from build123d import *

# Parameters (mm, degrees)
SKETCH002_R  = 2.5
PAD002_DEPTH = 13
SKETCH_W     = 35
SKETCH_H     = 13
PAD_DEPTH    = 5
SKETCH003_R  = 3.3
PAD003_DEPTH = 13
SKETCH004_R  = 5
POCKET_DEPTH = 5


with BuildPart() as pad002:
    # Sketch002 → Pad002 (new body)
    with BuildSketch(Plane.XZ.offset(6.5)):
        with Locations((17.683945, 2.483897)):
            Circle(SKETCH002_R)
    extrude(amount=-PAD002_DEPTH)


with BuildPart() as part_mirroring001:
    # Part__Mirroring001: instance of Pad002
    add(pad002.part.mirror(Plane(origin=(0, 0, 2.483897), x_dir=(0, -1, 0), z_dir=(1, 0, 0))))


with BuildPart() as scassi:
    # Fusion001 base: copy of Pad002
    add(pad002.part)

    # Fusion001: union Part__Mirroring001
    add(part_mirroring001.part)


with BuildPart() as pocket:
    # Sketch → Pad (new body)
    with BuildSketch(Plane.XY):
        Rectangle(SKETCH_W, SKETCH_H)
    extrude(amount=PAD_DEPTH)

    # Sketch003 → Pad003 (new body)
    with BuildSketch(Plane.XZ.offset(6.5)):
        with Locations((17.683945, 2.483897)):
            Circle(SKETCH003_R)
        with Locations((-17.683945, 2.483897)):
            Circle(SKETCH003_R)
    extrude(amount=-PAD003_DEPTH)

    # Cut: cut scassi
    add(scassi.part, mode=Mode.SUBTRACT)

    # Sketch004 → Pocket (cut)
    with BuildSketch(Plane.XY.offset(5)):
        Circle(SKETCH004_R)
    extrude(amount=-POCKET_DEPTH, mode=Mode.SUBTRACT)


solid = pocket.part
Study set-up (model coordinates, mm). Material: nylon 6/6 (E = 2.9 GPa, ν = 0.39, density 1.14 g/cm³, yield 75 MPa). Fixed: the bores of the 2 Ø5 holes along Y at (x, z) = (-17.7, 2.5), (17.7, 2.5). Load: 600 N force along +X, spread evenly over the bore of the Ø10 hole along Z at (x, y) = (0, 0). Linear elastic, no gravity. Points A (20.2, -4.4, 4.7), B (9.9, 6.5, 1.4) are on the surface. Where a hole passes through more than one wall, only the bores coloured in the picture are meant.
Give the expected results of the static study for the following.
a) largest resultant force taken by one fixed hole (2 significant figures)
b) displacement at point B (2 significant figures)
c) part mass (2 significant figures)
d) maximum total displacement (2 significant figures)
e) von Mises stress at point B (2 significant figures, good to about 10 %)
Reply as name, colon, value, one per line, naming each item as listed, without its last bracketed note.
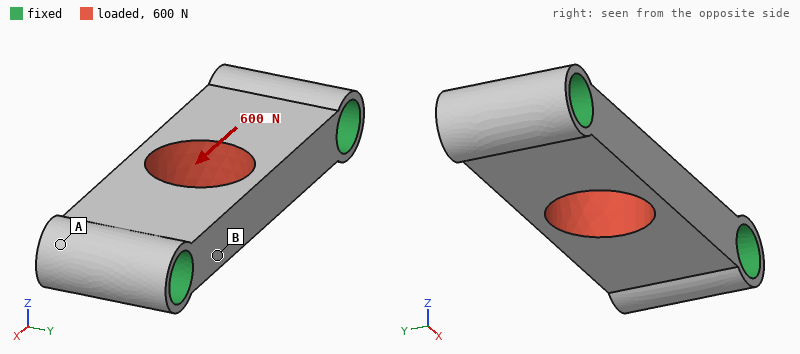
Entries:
largest resultant force taken by one fixed hole: 300 N
displacement at point B: 10 µm
part mass: 2.2 g
maximum total displacement: 27 µm
von Mises stress at point B: 4.8 MPa
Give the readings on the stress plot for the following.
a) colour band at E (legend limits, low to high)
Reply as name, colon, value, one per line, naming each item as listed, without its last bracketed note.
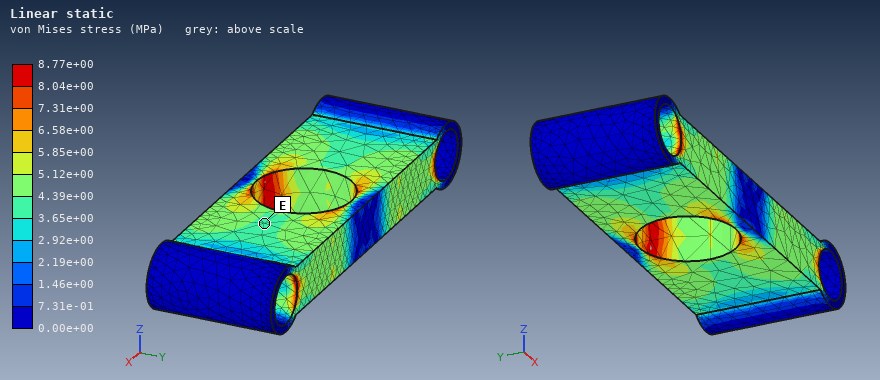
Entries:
colour band at E: 3.65e+00 to 4.39e+00 MPa
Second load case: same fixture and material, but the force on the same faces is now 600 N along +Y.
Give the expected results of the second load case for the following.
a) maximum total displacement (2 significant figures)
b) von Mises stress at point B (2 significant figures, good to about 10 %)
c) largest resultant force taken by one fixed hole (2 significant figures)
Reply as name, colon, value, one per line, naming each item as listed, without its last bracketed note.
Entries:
maximum total displacement: 0.13 mm
von Mises stress at point B: 4.8 MPa
largest resultant force taken by one fixed hole: 300 N
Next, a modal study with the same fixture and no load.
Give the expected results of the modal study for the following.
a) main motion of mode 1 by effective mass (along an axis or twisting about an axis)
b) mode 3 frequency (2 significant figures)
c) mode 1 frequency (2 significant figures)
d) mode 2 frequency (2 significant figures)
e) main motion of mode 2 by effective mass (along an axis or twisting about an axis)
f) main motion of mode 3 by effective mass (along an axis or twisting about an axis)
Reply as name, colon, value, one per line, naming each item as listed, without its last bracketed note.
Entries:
main motion of mode 1 by effective mass: along Z
mode 3 frequency: 15 kHz
mode 1 frequency: 8000 Hz
mode 2 frequency: 11 kHz
main motion of mode 2 by effective mass: twisting about X
main motion of mode 3 by effective mass: along Y
